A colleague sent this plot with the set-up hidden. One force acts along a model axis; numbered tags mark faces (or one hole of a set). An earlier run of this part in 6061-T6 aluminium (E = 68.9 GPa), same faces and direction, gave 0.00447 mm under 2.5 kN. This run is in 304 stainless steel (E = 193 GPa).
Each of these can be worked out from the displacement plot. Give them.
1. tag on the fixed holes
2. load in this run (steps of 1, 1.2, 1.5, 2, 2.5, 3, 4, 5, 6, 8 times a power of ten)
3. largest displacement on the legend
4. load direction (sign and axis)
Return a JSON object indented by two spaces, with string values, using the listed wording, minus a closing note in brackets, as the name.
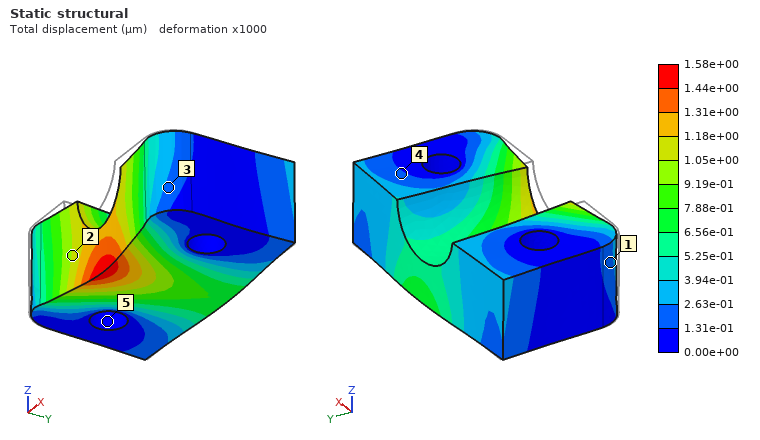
{
  "tag on the fixed holes": "5",
  "load in this run": "2.5 kN",
  "largest displacement on the legend": "1.58e+00 µm",
  "load direction": "+Y"
}
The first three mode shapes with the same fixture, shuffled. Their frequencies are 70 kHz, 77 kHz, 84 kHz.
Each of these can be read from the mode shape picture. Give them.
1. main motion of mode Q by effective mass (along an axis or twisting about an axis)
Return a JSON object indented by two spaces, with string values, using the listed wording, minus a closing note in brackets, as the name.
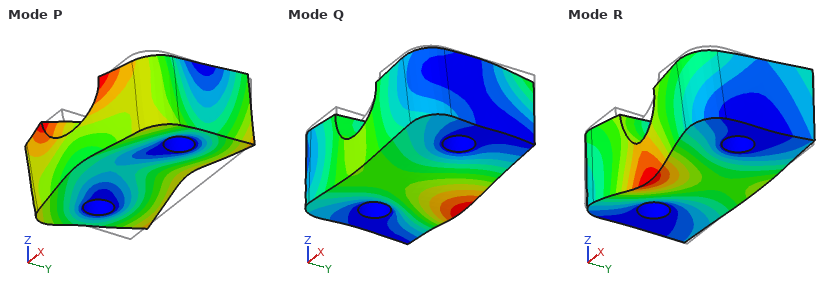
{
  "main motion of mode Q by effective mass": "along Z"
}
